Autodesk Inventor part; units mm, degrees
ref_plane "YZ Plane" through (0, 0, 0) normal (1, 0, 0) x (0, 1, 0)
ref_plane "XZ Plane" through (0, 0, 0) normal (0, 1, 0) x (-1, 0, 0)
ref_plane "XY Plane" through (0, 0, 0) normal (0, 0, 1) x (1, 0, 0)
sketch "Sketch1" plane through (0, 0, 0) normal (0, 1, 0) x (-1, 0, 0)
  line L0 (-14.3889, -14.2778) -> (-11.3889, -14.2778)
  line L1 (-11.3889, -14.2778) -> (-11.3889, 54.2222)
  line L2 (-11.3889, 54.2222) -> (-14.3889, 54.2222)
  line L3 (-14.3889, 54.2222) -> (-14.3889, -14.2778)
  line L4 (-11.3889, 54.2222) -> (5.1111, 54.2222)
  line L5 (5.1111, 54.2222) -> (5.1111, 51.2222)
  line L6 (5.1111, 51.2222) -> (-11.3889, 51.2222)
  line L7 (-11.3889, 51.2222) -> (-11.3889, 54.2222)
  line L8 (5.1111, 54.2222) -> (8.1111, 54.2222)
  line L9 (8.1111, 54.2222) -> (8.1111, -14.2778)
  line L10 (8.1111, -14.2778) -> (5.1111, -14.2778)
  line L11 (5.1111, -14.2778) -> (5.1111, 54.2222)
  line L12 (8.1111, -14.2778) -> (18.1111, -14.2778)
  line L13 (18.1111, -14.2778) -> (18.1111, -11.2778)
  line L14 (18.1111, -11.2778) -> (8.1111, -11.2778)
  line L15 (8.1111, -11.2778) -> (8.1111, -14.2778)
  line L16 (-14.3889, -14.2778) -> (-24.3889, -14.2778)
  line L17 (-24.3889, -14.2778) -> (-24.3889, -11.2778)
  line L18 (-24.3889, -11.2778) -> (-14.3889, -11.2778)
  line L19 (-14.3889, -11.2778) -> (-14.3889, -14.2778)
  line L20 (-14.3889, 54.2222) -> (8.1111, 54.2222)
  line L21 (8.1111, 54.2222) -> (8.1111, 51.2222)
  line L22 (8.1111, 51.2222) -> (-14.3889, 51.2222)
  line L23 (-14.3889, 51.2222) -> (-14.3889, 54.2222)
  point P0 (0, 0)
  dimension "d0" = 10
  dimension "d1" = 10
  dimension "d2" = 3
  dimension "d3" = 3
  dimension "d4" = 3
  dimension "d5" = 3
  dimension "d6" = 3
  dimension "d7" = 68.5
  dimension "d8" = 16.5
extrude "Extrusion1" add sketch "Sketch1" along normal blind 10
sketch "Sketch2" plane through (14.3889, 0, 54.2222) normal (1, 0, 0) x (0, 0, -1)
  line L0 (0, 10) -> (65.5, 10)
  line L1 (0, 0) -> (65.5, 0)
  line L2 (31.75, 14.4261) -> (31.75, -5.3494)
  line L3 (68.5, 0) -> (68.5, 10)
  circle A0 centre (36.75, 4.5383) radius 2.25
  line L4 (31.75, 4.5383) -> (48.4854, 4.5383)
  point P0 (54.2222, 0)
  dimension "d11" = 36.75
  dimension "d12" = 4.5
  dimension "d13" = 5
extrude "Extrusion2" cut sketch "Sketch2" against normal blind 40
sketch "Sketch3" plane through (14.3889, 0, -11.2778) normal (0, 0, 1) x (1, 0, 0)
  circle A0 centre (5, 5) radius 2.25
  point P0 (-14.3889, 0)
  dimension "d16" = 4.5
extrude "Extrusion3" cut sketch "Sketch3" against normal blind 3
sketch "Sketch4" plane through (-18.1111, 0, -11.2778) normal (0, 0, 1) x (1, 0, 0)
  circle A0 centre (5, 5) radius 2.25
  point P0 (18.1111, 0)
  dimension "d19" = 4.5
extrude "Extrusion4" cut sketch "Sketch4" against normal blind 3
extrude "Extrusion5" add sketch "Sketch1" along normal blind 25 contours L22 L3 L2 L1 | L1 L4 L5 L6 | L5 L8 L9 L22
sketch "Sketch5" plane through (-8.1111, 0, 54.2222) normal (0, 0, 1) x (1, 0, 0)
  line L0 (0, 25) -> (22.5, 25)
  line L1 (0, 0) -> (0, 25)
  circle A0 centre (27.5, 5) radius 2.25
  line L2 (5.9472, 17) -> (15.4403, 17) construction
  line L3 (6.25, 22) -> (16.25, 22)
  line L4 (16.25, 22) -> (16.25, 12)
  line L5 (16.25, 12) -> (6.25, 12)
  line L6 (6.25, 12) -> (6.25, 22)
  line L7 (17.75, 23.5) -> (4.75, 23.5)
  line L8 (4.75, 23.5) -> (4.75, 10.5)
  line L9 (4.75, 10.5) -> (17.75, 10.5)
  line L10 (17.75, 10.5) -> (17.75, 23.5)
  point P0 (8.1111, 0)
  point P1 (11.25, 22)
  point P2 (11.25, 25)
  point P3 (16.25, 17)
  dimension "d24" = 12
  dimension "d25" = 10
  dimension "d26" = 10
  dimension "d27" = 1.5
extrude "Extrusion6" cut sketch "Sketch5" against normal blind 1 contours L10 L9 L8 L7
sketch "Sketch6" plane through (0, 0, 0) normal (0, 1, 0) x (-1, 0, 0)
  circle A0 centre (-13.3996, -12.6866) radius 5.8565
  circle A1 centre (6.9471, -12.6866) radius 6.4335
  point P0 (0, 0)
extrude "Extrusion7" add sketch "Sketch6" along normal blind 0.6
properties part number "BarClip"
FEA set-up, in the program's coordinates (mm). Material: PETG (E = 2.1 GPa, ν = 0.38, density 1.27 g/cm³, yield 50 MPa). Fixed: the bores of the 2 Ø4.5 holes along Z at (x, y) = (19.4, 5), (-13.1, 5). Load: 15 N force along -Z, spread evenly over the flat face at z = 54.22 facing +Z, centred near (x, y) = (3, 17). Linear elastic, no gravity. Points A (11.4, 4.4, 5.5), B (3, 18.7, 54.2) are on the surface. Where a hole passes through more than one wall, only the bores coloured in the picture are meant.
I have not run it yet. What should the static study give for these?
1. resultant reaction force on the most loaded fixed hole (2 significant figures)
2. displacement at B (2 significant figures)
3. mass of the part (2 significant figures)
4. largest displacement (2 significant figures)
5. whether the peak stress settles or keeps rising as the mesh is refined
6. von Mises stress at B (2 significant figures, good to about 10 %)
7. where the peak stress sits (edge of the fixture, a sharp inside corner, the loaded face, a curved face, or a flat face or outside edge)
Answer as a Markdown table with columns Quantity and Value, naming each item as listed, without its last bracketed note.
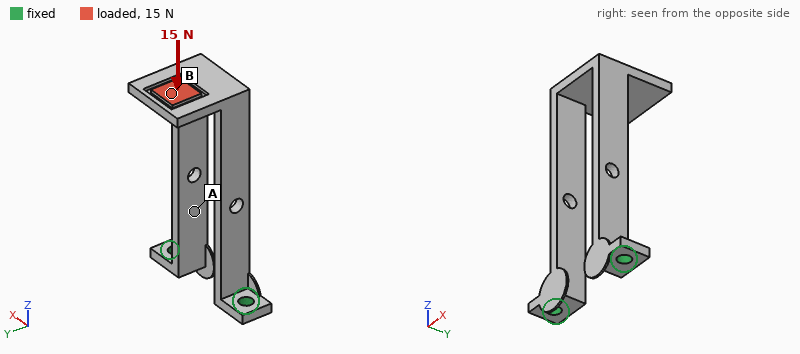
| Quantity | Value |
|---|---|
| resultant reaction force on the most loaded fixed hole | 7.5 N |
| displacement at B | 0.75 mm |
| mass of the part | 7.7 g |
| largest displacement | 0.84 mm |
| whether the peak stress settles or keeps rising as the mesh is refined | keeps rising |
| von Mises stress at B | 1.6 MPa |
| where the peak stress sits | edge of the fixture |
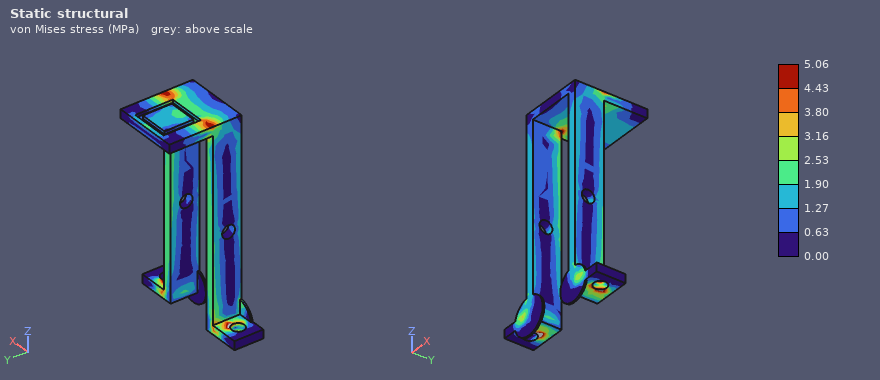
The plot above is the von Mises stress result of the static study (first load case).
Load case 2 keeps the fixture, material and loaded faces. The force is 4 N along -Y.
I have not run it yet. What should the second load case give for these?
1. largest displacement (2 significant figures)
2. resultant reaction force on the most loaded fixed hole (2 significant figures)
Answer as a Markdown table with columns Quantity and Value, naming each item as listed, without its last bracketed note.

| Quantity | Value |
|---|---|
| largest displacement | 0.86 mm |
| resultant reaction force on the most loaded fixed hole | 2.0 N |
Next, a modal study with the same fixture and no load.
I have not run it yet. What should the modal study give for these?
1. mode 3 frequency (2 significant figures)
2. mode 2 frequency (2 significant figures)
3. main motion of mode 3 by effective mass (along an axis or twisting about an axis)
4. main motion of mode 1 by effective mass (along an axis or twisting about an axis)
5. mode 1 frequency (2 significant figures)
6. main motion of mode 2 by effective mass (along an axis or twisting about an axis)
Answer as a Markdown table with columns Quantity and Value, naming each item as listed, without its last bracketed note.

| Quantity | Value |
|---|---|
| mode 3 frequency | 410 Hz |
| mode 2 frequency | 200 Hz |
| main motion of mode 3 by effective mass | twisting about Z |
| main motion of mode 1 by effective mass | along X |
| mode 1 frequency | 160 Hz |
| main motion of mode 2 by effective mass | along Y |
